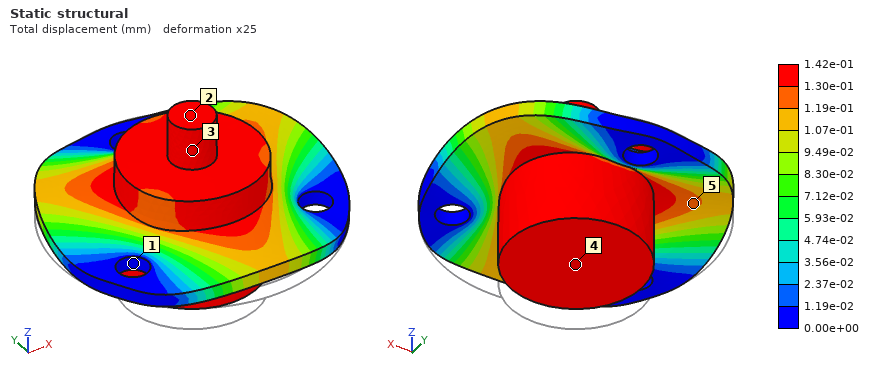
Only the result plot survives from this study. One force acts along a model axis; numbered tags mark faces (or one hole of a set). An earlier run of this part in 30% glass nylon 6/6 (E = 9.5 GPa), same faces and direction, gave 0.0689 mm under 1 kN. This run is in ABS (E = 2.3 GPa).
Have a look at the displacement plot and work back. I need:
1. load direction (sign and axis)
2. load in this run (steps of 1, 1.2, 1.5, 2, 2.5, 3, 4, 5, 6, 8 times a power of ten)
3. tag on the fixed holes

+Z
500 N
1
